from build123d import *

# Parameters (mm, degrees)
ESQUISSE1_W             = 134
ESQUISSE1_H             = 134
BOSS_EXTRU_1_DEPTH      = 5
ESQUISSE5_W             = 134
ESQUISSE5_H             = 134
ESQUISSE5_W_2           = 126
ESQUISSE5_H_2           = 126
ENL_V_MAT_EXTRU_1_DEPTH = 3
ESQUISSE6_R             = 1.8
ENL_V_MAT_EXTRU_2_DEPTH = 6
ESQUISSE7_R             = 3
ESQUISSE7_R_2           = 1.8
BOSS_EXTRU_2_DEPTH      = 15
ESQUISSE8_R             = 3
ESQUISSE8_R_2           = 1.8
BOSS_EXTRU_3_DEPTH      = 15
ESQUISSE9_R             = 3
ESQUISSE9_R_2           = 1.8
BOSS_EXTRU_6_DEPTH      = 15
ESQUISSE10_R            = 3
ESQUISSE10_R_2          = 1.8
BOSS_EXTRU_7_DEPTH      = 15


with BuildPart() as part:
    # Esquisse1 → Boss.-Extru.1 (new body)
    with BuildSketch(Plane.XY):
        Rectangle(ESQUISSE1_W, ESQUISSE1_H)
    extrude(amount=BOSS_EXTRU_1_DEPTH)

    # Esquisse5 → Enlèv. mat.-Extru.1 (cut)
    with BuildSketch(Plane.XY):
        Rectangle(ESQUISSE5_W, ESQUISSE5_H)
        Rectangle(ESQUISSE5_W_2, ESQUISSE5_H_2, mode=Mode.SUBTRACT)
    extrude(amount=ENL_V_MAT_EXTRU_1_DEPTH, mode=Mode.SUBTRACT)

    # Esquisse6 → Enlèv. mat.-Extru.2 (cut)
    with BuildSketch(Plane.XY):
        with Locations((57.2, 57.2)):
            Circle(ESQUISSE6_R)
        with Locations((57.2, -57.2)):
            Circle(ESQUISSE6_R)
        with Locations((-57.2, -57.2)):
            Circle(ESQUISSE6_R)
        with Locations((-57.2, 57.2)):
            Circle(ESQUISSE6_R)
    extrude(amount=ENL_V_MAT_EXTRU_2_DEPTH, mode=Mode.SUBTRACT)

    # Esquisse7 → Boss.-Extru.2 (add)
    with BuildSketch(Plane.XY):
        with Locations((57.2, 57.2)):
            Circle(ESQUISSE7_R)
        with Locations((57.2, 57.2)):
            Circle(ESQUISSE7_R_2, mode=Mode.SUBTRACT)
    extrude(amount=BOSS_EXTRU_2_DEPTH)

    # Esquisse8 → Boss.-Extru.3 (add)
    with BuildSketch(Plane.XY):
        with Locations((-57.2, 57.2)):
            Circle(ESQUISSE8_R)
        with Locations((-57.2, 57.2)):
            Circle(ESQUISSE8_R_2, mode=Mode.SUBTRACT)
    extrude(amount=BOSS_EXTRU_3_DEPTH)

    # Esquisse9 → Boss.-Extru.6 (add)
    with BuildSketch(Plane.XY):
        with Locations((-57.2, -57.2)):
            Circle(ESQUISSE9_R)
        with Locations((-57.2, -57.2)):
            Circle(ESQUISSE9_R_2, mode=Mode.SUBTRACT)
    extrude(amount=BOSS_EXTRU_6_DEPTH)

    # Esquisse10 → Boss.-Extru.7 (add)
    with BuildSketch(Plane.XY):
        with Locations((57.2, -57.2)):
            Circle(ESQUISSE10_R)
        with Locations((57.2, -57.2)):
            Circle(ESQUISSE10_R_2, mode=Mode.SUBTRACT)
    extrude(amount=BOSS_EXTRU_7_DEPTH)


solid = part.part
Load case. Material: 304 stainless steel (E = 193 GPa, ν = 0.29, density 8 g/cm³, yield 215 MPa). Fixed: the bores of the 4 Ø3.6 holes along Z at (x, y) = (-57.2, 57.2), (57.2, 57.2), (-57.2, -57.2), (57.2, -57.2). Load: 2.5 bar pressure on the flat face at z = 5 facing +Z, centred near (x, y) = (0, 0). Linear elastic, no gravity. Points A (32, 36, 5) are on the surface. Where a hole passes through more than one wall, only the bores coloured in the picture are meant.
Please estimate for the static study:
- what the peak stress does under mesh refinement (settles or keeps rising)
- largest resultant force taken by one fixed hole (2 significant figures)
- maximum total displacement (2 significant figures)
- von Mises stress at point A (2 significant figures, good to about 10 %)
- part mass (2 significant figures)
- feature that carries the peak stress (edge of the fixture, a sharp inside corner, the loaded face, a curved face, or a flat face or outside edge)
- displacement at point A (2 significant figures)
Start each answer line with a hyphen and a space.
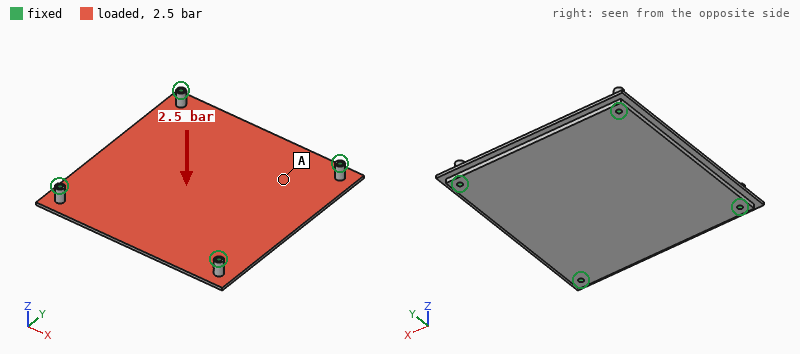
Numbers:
- keeps rising
- 1.1 kN
- 0.18 mm
- 24 MPa
- 670 g
- edge of the fixture
- 0.100 mm
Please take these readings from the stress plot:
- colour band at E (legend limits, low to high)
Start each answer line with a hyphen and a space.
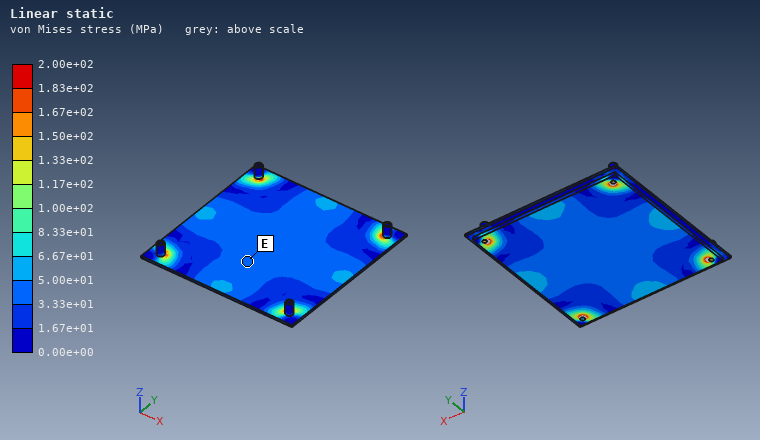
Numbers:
- 3.33e+01 to 5.00e+01 MPa
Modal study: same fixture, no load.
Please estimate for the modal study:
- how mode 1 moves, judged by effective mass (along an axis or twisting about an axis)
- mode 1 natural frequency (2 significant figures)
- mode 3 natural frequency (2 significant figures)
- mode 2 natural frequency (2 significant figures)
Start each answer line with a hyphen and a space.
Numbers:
- along Z
- 1100 Hz
- 2000 Hz
- 2000 Hz
